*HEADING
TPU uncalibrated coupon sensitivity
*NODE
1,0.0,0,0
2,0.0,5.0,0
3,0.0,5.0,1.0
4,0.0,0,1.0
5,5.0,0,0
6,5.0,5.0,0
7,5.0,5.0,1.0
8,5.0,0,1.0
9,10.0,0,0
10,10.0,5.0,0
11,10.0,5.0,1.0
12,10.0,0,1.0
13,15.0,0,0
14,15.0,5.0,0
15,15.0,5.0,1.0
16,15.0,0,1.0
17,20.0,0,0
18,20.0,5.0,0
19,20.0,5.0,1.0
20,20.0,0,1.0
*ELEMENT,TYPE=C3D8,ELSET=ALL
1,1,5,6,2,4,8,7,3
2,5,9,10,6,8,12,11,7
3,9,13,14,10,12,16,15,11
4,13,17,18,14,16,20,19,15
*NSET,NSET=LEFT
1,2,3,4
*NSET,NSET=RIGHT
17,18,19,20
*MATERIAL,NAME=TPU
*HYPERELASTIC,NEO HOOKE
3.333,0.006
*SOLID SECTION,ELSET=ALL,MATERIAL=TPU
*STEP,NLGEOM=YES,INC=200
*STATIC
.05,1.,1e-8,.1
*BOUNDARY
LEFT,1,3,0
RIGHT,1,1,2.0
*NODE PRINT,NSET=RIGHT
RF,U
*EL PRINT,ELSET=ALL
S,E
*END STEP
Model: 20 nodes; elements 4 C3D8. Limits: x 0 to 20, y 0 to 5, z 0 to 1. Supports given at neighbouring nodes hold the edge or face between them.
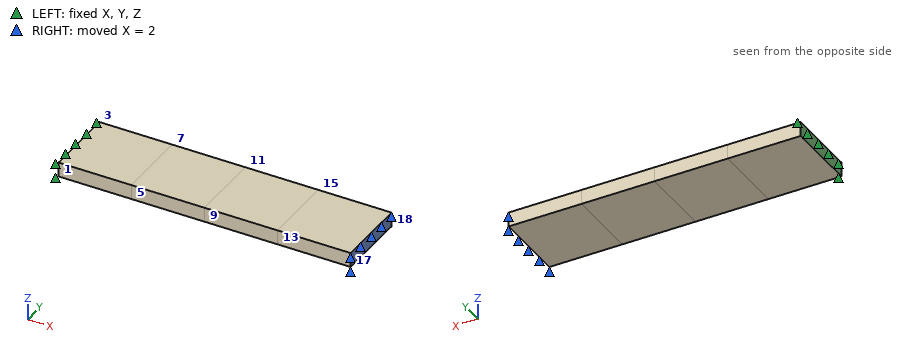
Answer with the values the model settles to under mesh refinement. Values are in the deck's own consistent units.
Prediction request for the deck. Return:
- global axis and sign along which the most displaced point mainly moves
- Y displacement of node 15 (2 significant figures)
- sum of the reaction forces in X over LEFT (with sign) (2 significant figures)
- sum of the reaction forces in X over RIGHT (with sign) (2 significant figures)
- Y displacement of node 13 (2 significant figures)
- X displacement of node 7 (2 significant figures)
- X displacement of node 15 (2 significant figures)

+X
-0.12
-9.2
9.2
0.12
0.48
1.5
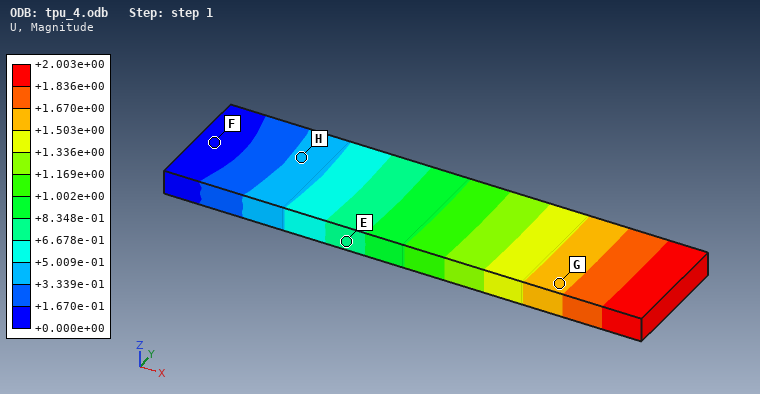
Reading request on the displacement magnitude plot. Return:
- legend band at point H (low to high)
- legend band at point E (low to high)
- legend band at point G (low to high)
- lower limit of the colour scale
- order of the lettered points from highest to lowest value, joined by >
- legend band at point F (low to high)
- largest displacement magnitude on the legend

+3.339e-01 to +5.009e-01
+6.678e-01 to +8.348e-01
+1.503e+00 to +1.670e+00
+0.000e+00
G > E > H > F
+0.000e+00 to +1.670e-01
+2.003e+00
